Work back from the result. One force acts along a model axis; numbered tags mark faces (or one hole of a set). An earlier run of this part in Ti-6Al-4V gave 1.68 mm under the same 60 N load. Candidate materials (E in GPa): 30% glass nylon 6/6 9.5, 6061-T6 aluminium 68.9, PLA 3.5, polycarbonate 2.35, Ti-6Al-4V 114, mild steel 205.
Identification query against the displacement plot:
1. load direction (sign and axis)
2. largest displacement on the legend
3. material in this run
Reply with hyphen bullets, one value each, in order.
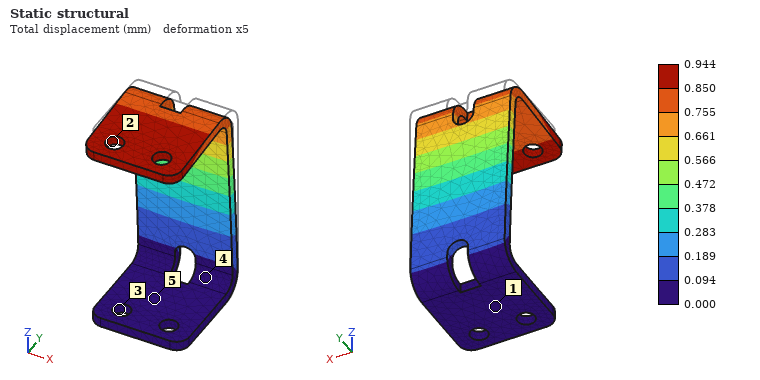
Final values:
- -Y
- 0.944 mm
- mild steel
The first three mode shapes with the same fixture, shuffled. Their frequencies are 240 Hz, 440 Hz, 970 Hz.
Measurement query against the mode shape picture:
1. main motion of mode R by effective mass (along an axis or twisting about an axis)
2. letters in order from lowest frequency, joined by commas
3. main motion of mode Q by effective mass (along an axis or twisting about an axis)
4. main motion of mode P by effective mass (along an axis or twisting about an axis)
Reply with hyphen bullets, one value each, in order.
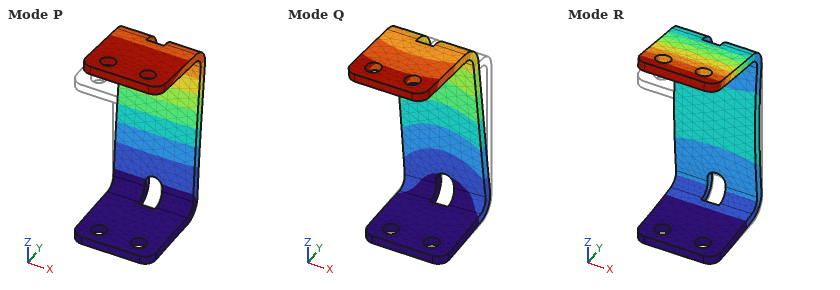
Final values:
- along Z
- P, Q, R
- along X
- along Y
